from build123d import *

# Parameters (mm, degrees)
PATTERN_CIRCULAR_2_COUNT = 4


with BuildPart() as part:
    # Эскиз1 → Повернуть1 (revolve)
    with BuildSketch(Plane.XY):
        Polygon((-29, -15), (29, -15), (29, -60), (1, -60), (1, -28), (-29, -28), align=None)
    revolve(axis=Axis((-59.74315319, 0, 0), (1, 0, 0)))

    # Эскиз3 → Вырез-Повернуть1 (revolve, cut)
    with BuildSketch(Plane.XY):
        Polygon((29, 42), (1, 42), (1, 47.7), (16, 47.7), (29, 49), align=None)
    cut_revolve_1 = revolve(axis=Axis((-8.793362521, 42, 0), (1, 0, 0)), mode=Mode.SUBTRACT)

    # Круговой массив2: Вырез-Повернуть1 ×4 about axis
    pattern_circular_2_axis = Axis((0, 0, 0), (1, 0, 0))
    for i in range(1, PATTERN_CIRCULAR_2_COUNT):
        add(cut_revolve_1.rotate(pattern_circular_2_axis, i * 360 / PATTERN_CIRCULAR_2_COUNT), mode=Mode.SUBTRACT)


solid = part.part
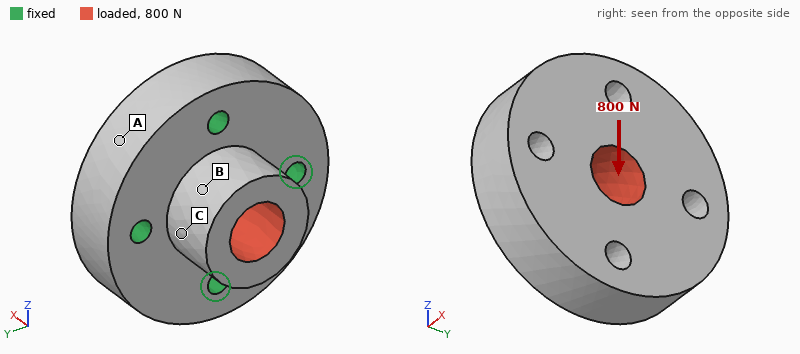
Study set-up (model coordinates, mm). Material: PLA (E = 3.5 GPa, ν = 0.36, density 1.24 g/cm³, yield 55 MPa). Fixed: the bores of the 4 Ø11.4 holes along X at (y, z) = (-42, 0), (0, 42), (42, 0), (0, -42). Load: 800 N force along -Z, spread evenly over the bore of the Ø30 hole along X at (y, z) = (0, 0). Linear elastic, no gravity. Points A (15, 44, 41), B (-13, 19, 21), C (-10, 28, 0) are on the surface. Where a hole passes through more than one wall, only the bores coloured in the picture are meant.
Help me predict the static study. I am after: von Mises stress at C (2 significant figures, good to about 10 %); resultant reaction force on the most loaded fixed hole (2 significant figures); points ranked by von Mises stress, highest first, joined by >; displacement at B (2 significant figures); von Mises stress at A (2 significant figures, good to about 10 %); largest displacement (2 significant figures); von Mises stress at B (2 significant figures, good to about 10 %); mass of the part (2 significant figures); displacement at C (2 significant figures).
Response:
0.30 MPa
250 N
C > B > A
7.6 µm
0.093 MPa
12 µm
0.20 MPa
420 g
5.9 µm
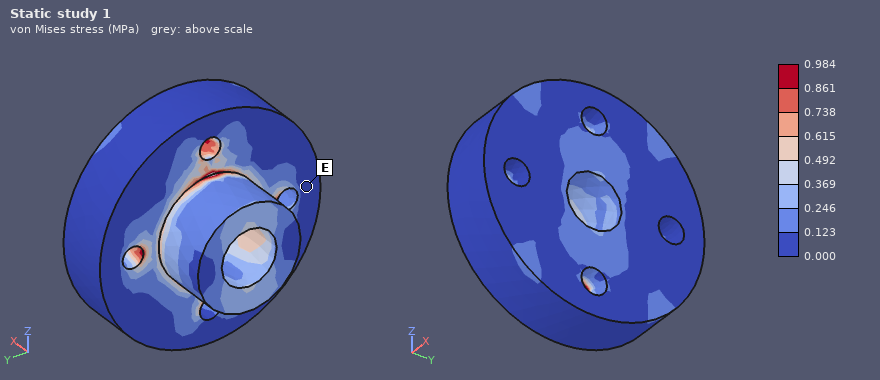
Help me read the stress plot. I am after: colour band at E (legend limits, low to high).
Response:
0.000 to 0.123 MPa
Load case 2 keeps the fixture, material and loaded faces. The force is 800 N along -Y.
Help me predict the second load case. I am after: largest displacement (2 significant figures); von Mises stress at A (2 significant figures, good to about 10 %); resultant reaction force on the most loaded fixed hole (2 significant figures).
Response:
12 µm
0.099 MPa
250 N
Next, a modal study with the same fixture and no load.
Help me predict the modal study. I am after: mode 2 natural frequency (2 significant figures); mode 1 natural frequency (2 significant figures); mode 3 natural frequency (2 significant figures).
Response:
4000 Hz
3900 Hz
4000 Hz
